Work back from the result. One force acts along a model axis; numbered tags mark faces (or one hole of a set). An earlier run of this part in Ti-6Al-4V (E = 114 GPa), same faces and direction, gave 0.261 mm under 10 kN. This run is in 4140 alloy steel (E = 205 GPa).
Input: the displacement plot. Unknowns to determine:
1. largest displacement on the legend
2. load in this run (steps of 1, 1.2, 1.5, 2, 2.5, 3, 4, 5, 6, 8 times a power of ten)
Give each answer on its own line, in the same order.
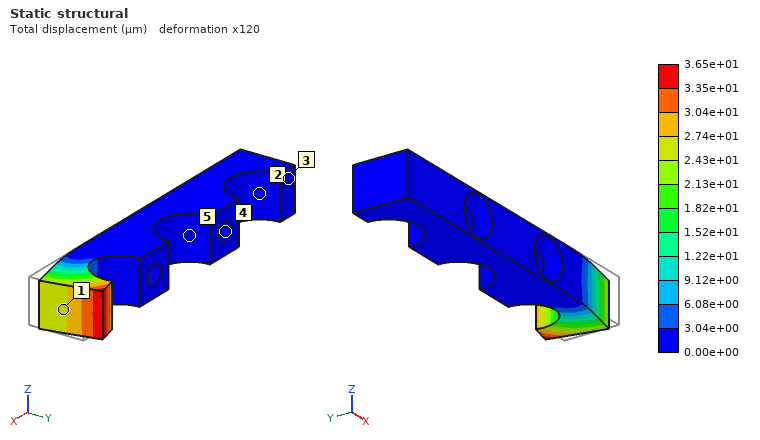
3.65e+01 µm
2.5 kN
